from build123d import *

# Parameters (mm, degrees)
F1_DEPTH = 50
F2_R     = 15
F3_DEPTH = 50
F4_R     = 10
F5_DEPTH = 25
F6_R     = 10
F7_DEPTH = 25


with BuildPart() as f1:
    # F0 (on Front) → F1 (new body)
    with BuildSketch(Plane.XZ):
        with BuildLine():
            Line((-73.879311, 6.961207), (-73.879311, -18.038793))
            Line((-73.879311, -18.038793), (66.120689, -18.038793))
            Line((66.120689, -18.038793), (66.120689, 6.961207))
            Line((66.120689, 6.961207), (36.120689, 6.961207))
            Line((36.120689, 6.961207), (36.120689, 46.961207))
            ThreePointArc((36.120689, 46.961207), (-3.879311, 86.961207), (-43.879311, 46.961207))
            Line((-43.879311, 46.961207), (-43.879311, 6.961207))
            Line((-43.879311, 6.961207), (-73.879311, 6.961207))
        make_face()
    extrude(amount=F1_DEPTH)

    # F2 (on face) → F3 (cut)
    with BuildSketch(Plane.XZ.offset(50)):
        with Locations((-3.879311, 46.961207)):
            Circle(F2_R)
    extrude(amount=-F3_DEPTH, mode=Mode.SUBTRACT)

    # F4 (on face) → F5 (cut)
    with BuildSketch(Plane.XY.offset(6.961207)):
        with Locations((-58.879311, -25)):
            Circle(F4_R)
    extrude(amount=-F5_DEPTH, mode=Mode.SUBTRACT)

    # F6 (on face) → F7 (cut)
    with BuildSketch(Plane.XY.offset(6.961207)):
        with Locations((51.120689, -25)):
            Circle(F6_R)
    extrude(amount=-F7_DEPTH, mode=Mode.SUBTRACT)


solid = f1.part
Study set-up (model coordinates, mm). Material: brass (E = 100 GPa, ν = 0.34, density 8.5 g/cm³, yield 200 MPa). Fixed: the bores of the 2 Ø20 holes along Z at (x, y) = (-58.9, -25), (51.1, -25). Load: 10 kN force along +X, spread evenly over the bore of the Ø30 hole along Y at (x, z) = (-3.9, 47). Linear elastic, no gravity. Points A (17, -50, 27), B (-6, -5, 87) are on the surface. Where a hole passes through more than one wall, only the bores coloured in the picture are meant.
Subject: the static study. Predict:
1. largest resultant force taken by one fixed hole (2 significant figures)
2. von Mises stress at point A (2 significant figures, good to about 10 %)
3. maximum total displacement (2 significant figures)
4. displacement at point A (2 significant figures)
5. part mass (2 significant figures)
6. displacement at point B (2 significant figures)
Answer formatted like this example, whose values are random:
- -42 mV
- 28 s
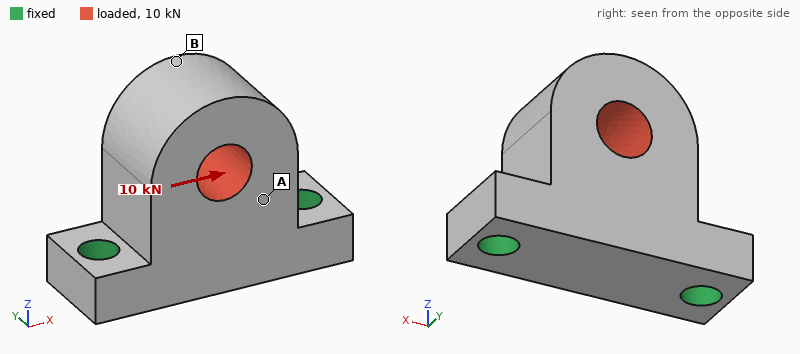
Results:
- 7.6 kN
- 4.2 MPa
- 14 µm
- 4.7 µm
- 3.5 kg
- 14 µm
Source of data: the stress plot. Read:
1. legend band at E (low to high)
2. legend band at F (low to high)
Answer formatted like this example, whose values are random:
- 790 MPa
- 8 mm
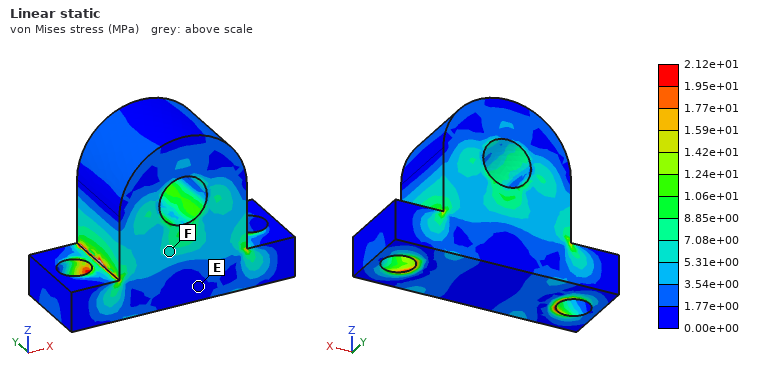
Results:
- 0.00e+00 to 1.77e+00 MPa
- 5.31e+00 to 7.08e+00 MPa
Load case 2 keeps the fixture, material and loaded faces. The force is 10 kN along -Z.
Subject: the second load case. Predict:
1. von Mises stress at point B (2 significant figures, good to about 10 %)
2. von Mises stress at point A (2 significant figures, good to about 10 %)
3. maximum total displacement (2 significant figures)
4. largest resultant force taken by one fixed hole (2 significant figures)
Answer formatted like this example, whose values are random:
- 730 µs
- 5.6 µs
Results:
- 1.9 MPa
- 3.2 MPa
- 5.2 µm
- 5.3 kN
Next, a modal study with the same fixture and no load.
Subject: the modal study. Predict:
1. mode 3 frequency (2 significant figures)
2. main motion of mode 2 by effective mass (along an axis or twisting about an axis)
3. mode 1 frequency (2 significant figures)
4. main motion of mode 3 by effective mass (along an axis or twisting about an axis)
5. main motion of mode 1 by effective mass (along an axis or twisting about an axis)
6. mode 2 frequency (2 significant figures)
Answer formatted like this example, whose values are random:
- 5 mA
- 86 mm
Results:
- 4800 Hz
- along X
- 1600 Hz
- along Z
- along Y
- 3400 Hz
